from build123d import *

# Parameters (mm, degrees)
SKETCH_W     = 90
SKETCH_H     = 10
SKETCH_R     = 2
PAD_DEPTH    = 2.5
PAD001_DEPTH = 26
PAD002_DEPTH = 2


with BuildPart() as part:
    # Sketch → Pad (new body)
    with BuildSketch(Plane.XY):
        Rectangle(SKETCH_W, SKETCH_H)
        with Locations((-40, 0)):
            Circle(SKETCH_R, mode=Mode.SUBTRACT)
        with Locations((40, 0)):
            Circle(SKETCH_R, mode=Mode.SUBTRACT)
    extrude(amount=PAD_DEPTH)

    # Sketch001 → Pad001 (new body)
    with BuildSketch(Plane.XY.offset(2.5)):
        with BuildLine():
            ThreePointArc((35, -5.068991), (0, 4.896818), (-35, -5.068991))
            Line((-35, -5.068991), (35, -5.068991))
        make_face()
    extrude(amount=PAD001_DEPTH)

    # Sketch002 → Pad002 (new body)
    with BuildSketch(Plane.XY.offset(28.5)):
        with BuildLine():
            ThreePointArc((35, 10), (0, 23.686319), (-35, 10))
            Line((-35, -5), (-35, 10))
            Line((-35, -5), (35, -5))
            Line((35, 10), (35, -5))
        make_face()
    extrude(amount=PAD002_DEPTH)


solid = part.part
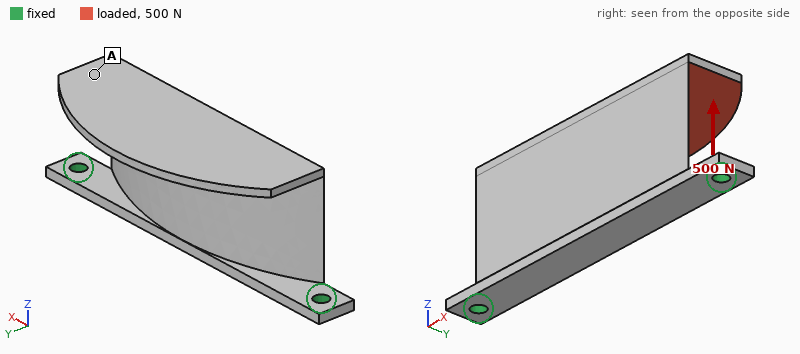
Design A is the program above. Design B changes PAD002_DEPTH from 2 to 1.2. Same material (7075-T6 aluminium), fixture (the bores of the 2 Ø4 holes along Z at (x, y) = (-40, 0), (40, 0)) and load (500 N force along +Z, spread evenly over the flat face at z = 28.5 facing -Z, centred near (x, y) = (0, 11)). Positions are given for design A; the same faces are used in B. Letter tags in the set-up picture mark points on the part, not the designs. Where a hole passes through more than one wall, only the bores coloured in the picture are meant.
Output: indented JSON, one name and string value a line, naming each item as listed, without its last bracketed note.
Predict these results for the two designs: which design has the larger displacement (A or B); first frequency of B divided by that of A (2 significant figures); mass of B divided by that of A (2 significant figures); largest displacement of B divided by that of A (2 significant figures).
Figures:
{
  "which design has the larger displacement": "B",
  "first frequency of B divided by that of A": "1.1",
  "mass of B divided by that of A": "0.92",
  "largest displacement of B divided by that of A": "1.3"
}
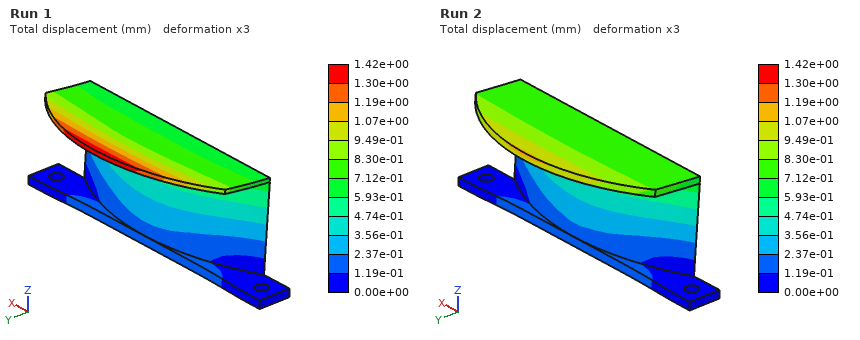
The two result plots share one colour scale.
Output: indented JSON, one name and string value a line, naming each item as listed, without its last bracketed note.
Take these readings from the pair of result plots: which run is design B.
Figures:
{
  "which run is design B": "Run 1"
}
